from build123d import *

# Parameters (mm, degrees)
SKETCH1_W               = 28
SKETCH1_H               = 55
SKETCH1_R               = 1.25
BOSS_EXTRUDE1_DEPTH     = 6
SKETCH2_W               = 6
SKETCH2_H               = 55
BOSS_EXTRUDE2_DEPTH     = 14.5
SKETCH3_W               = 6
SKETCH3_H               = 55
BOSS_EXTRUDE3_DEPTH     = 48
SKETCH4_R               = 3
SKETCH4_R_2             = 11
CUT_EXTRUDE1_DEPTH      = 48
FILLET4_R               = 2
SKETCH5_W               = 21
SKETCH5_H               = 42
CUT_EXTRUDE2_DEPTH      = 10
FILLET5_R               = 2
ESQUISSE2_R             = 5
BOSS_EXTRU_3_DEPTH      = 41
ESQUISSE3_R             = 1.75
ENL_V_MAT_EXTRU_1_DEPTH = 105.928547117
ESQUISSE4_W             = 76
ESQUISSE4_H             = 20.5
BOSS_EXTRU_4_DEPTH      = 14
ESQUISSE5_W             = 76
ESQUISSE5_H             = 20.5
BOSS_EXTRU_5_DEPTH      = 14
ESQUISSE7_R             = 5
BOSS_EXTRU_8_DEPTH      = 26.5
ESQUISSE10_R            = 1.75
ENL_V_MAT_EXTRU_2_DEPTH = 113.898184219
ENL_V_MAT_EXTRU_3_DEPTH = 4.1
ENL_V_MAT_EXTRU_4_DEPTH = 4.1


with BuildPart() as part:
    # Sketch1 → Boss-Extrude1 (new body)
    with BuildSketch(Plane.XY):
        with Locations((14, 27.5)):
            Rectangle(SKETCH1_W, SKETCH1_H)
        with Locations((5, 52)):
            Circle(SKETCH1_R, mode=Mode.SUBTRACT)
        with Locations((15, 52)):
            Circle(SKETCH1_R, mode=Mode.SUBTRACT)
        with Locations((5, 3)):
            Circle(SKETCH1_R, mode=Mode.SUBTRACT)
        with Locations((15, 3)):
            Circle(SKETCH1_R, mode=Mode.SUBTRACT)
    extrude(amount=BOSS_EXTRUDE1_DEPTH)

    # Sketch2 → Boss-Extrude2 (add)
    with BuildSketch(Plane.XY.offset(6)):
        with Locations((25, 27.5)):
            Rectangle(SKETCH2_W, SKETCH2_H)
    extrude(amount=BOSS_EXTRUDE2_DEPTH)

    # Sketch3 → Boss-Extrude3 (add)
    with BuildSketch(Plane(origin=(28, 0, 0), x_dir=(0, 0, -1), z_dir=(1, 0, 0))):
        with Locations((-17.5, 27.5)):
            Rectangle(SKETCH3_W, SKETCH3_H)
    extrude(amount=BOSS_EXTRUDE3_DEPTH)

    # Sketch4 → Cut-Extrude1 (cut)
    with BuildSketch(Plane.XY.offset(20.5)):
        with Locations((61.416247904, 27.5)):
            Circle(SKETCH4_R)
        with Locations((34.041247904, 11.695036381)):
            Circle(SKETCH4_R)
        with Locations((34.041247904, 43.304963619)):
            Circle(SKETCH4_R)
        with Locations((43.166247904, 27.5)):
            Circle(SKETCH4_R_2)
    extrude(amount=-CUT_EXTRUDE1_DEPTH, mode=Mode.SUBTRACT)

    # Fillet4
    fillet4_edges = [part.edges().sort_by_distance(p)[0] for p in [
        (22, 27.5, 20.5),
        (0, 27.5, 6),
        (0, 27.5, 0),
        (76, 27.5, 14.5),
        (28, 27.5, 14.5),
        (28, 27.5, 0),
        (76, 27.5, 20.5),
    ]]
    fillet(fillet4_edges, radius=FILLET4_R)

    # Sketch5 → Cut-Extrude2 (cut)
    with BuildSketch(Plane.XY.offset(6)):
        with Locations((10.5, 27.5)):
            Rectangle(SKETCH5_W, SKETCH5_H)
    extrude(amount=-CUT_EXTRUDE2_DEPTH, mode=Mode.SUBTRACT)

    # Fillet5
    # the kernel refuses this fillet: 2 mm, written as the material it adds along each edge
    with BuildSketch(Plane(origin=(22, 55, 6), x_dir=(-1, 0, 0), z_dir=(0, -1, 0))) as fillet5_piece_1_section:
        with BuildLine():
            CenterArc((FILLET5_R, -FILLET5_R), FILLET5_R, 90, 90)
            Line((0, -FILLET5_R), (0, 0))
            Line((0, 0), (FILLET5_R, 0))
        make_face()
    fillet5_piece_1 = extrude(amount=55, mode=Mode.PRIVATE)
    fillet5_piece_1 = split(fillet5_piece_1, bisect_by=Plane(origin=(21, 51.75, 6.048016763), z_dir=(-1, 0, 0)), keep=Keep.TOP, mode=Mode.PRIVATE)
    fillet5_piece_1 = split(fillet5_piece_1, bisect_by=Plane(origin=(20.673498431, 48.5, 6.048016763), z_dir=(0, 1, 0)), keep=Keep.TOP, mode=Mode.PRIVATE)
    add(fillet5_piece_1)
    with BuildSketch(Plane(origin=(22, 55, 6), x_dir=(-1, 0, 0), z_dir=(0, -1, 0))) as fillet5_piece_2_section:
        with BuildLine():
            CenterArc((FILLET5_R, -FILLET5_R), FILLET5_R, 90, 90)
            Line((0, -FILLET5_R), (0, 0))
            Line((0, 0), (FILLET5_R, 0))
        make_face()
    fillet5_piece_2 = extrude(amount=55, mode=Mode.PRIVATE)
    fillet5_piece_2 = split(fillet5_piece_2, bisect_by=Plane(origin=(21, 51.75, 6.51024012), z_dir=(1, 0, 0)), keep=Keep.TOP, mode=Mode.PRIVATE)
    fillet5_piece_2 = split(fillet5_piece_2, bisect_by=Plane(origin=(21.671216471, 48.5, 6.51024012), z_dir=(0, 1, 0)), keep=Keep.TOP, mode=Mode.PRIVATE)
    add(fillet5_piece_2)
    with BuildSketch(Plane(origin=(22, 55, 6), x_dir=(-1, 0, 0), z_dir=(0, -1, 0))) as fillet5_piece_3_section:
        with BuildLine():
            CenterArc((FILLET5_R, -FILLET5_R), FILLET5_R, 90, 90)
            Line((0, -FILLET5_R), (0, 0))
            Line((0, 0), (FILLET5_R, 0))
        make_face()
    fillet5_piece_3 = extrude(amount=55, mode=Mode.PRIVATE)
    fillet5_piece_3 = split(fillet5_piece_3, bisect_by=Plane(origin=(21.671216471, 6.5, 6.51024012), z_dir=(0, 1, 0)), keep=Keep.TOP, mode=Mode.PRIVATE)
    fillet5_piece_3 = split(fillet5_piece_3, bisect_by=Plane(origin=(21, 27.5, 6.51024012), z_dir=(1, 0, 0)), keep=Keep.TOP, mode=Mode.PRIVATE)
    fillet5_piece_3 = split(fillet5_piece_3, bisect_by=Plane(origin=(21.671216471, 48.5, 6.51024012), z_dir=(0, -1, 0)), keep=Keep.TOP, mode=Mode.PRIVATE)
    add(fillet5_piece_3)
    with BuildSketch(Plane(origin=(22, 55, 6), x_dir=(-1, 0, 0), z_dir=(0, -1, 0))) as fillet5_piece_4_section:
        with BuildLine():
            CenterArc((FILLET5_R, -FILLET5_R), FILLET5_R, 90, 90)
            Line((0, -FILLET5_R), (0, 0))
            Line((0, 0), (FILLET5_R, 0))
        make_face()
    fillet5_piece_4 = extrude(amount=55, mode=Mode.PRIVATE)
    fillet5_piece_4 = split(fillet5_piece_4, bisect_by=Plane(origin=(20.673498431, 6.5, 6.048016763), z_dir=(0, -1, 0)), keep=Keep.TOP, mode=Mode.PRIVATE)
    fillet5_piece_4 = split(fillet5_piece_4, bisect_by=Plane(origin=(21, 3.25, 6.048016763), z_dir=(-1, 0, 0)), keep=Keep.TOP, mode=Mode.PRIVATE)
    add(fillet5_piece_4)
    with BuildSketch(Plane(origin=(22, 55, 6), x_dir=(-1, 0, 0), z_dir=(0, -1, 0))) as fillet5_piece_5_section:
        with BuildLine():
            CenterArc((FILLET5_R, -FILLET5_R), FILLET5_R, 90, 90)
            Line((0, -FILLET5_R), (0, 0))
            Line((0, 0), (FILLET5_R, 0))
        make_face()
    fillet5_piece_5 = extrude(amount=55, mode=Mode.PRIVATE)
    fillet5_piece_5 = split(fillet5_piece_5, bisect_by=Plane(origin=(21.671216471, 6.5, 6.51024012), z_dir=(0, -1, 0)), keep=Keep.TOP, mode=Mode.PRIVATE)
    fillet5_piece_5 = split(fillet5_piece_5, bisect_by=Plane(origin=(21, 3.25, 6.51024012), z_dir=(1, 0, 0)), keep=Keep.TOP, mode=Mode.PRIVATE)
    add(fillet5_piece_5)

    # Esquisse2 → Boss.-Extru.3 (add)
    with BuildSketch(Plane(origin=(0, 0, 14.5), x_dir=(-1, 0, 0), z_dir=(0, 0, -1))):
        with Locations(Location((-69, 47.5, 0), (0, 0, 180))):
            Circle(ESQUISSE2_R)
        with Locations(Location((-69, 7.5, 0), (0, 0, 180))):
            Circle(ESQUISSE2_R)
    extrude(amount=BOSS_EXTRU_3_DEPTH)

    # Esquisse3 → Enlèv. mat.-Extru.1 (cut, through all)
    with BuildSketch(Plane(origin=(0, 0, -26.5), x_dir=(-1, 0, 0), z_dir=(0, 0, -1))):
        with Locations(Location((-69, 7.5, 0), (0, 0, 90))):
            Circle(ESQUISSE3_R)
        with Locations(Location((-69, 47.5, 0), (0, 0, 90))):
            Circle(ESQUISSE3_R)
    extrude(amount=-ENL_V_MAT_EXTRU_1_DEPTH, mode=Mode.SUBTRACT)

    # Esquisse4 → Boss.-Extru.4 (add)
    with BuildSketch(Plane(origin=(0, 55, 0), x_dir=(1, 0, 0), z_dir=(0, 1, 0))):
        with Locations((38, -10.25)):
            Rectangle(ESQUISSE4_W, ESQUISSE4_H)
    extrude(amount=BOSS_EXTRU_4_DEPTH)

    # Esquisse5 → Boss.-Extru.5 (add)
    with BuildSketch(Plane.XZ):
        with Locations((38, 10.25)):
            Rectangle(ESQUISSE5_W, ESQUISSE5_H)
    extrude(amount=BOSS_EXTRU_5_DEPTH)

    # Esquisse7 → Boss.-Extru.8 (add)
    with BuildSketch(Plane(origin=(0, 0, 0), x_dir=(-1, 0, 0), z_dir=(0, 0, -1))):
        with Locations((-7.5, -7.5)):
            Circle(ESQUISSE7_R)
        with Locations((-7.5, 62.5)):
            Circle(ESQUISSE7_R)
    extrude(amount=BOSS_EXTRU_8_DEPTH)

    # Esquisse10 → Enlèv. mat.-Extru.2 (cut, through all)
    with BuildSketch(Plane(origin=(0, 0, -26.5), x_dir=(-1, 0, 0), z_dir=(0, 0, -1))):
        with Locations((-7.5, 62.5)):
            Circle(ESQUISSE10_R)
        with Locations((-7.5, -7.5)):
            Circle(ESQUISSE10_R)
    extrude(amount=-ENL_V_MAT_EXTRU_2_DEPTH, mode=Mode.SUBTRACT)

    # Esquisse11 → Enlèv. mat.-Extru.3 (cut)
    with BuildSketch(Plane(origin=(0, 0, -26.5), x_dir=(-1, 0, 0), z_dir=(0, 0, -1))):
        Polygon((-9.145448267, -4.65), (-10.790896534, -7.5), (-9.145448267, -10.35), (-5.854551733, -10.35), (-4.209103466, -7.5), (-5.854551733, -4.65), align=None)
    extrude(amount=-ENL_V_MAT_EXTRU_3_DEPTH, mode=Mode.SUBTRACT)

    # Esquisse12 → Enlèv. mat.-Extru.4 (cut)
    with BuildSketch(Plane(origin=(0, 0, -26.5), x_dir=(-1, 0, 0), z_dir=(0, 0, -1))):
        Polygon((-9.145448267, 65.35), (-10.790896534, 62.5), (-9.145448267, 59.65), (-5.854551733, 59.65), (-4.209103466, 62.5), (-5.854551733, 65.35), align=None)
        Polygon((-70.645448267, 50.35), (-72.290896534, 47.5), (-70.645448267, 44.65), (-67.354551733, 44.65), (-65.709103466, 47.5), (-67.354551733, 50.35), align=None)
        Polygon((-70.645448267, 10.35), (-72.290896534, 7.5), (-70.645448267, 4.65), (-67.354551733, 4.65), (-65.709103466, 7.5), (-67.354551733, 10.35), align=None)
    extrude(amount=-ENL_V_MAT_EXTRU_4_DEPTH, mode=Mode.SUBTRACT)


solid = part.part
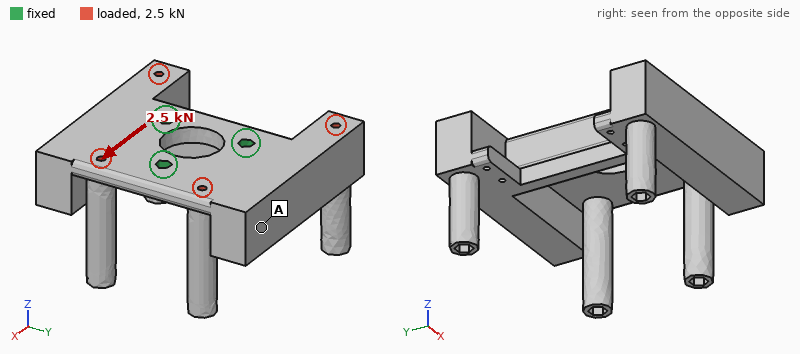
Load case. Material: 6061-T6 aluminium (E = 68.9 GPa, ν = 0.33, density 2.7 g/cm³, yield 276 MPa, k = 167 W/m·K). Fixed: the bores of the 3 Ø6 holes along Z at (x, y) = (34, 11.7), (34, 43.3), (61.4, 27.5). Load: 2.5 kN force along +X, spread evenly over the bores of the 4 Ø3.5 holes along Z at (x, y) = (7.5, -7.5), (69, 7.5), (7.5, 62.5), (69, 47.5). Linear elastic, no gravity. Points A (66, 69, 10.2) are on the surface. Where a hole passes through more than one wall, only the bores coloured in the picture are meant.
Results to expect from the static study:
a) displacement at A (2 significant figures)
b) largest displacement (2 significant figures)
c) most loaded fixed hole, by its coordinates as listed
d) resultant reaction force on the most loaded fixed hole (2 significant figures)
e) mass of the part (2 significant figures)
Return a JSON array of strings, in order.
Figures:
["0.042 mm", "0.27 mm", "(61.4, 27.5)", "1.1 kN", "200 g"]
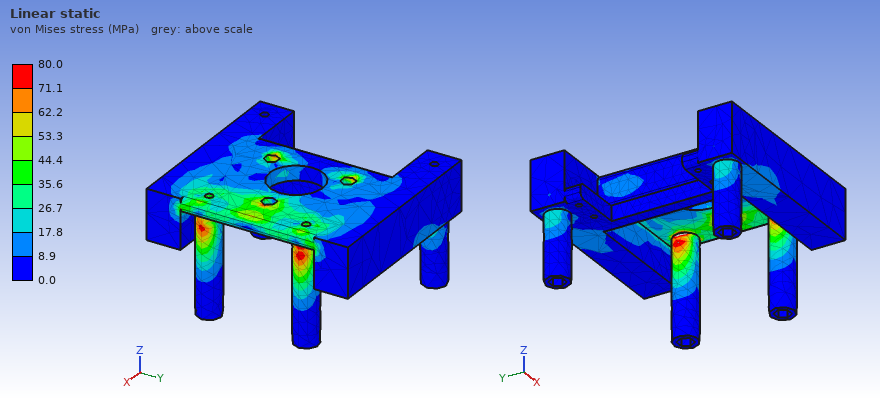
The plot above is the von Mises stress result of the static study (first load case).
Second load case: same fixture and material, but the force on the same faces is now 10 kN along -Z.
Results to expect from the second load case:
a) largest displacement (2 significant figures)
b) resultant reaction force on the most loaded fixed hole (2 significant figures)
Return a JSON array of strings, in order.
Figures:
["0.16 mm", "5.1 kN"]
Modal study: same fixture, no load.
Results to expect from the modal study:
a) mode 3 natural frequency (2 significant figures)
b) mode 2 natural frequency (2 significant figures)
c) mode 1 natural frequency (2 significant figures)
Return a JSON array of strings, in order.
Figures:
["3300 Hz", "2400 Hz", "2400 Hz"]
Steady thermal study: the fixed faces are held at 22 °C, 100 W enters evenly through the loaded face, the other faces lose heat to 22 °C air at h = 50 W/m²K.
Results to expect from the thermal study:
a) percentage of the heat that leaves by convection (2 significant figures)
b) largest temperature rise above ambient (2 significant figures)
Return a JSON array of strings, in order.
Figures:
["19 %", "46 K"]
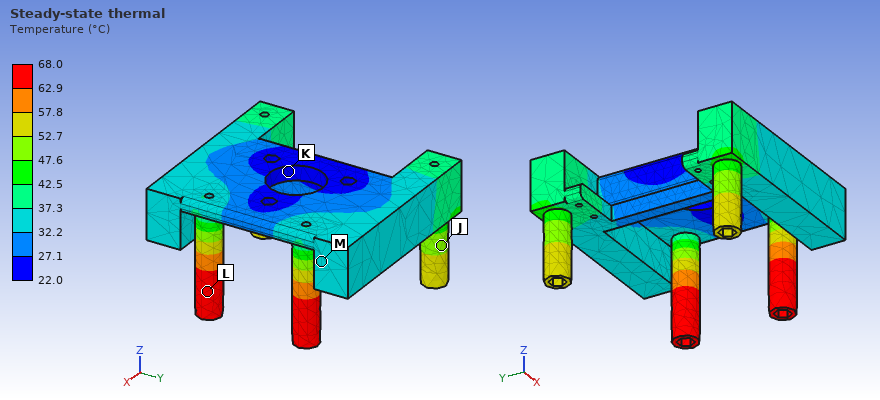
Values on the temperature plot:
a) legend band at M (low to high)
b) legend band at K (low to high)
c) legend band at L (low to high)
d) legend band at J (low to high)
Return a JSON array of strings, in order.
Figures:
["32.2 to 37.3 °C", "22.0 to 27.1 °C", "62.9 to 68.0 °C", "47.6 to 52.7 °C"]
